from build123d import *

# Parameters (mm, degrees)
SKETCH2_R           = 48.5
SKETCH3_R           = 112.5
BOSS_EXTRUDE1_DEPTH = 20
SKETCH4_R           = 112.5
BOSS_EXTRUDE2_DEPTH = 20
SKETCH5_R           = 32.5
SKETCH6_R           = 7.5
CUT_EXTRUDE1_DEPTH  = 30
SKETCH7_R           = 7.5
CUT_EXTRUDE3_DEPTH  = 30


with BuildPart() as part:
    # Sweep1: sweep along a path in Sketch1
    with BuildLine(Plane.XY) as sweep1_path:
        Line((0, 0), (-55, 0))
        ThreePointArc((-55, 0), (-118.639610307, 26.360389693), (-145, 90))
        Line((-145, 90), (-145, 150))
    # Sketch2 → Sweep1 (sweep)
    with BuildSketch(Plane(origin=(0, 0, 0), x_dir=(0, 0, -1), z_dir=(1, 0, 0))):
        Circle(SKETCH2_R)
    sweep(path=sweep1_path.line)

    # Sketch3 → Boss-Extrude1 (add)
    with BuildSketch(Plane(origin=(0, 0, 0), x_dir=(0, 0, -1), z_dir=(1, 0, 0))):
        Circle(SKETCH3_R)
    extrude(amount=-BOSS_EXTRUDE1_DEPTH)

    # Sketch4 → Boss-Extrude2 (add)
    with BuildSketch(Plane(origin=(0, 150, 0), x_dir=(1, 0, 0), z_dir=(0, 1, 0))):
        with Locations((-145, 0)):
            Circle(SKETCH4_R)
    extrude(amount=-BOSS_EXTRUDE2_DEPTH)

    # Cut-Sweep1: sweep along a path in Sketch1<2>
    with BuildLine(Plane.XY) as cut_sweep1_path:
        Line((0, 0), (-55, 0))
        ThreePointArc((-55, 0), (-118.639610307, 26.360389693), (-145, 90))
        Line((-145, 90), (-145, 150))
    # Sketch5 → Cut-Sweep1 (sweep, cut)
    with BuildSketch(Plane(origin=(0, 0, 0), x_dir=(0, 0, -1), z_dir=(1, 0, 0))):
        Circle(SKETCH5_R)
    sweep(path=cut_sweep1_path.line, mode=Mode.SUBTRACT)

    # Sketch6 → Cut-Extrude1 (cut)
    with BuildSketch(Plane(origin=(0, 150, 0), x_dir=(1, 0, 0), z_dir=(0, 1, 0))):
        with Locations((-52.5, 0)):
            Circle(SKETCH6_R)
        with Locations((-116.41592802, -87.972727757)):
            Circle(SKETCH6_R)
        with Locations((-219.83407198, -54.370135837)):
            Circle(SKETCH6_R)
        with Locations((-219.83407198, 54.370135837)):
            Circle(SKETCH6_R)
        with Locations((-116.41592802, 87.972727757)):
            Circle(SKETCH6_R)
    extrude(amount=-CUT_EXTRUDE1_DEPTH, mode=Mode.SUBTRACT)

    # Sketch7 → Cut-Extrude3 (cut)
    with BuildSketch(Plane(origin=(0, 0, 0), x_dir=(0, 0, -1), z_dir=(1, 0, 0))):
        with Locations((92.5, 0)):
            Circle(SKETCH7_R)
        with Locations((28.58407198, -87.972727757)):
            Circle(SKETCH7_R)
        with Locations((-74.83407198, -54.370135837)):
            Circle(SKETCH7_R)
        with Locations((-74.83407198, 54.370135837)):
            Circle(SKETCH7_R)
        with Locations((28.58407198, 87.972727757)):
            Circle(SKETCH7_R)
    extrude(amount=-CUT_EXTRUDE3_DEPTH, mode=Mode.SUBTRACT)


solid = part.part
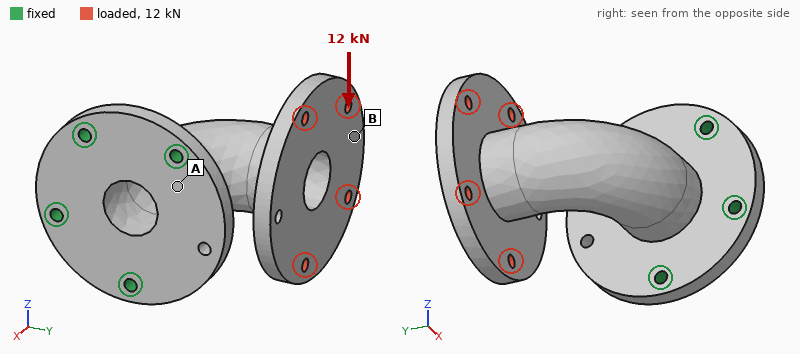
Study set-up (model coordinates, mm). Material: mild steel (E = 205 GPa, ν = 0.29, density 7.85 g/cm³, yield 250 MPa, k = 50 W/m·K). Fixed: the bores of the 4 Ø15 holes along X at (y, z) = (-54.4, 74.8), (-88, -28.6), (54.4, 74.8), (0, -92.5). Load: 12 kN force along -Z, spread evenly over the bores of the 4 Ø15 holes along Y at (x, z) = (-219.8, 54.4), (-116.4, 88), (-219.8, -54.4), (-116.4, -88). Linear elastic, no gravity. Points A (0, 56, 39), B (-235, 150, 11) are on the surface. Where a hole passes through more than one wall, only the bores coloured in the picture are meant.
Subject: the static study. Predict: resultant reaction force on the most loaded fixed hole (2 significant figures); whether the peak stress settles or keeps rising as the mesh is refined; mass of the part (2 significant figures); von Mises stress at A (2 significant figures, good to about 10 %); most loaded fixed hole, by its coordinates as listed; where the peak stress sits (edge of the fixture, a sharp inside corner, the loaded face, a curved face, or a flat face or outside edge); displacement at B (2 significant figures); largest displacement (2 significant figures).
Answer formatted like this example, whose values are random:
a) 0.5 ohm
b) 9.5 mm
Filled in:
a) 14 kN
b) keeps rising
c) 18 kg
d) 9.7 MPa
e) (0, -92.5)
f) edge of the fixture
g) 0.21 mm
h) 0.22 mm
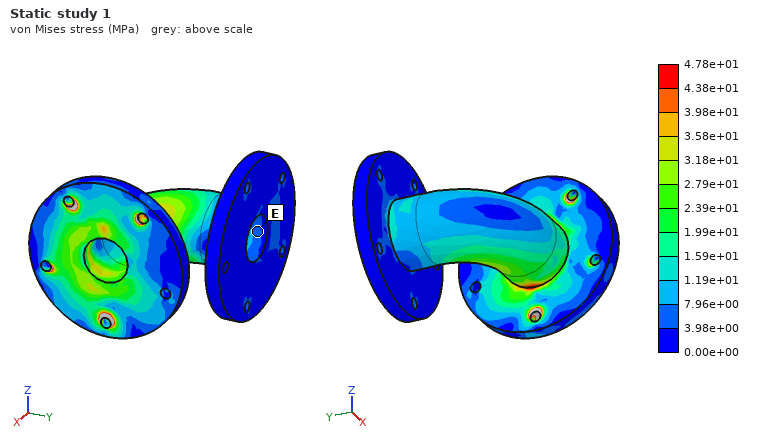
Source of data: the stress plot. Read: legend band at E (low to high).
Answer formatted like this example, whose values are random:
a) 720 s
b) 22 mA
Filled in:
a) 3.98e+00 to 7.96e+00 MPa
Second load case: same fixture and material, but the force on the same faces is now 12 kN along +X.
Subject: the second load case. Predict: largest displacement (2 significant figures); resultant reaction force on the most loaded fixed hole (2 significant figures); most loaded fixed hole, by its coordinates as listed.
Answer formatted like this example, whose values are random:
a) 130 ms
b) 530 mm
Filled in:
a) 0.27 mm
b) 15 kN
c) (54.4, 74.8)
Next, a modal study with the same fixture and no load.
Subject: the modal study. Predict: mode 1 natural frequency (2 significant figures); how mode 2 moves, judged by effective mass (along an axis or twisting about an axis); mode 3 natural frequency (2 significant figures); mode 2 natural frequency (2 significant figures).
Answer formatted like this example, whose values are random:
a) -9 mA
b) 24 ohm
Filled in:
a) 400 Hz
b) along Z
c) 1100 Hz
d) 520 Hz
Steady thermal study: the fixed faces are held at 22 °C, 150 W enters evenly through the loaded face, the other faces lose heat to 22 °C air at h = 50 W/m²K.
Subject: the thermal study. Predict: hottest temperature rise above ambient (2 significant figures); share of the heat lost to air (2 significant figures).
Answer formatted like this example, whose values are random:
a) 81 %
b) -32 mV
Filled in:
a) 41 K
b) 97 %
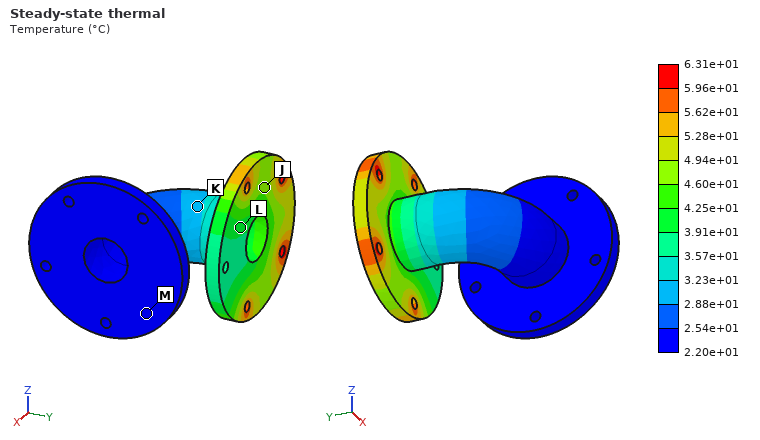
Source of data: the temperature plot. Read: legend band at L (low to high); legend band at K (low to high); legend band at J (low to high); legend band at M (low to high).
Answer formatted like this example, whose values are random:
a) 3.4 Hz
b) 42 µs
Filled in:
a) 3.91e+01 to 4.25e+01 °C
b) 2.88e+01 to 3.23e+01 °C
c) 4.60e+01 to 4.94e+01 °C
d) 2.20e+01 to 2.54e+01 °C
